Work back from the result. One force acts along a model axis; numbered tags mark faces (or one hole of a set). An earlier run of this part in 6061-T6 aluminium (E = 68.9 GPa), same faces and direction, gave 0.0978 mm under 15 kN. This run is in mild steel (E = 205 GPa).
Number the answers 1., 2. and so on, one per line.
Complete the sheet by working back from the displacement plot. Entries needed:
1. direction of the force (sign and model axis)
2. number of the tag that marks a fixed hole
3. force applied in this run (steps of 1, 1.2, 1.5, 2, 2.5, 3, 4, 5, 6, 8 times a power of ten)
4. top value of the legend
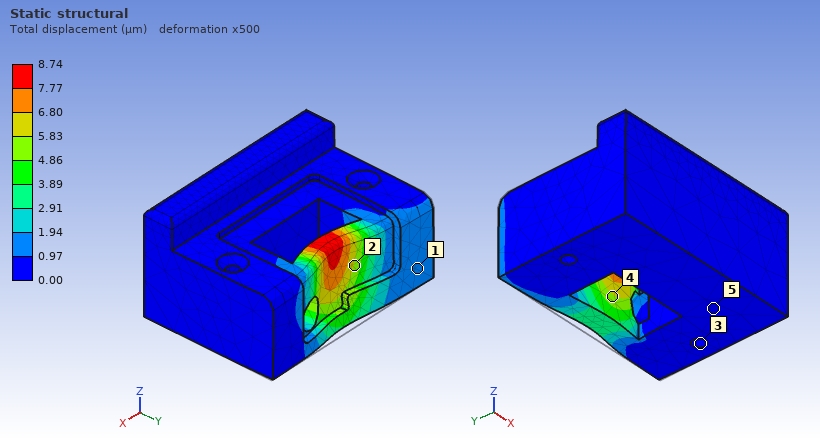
1. -Y
2. 3
3. 4 kN
4. 8.74 µm
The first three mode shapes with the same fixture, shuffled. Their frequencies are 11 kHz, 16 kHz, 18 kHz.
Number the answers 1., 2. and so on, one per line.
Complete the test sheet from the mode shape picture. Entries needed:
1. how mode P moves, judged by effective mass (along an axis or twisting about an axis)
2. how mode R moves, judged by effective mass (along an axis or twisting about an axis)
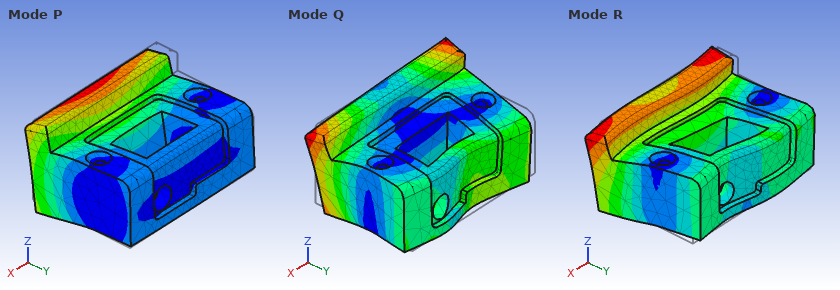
1. along Z
2. along X
